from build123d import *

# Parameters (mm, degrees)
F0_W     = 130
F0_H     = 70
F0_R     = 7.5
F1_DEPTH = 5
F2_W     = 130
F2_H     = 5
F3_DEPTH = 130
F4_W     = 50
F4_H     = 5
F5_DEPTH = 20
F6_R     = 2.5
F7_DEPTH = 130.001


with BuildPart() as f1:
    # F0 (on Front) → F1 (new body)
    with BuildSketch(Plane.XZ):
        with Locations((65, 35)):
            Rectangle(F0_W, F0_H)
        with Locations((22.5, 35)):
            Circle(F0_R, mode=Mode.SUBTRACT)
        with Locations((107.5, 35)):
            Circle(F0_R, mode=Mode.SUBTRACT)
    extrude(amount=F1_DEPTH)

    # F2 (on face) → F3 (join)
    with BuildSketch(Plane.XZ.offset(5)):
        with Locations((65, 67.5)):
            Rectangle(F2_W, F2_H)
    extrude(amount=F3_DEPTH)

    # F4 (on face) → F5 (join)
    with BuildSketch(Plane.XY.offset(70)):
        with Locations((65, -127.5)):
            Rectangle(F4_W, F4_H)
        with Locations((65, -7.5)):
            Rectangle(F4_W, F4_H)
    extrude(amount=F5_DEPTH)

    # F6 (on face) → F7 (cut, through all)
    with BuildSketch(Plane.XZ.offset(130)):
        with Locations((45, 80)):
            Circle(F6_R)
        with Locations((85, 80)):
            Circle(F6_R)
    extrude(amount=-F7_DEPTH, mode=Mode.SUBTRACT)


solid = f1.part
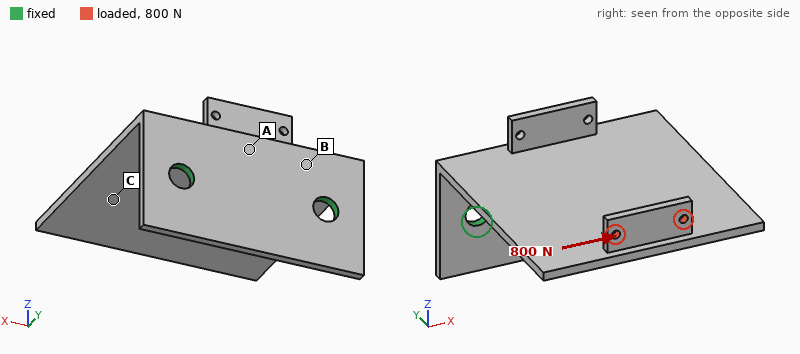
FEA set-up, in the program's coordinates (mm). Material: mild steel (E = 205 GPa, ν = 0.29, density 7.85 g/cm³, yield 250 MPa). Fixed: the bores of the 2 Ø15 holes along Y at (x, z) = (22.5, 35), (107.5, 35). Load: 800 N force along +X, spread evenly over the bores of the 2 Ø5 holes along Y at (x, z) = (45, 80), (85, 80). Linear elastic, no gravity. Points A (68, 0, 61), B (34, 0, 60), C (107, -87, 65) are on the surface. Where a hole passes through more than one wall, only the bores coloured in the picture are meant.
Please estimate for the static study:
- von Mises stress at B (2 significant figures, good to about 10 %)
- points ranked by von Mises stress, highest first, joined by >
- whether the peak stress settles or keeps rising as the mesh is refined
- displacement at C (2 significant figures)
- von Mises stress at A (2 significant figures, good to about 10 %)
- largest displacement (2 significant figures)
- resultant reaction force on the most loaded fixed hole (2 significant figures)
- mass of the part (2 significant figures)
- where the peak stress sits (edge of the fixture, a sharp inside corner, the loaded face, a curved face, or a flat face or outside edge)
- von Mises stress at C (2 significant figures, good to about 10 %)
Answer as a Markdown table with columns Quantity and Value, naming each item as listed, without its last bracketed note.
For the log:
| Quantity | Value |
|---|---|
| von Mises stress at B | 32 MPa |
| points ranked by von Mises stress, highest first, joined by > | B > A > C |
| whether the peak stress settles or keeps rising as the mesh is refined | keeps rising |
| displacement at C | 0.088 mm |
| von Mises stress at A | 19 MPa |
| largest displacement | 0.15 mm |
| resultant reaction force on the most loaded fixed hole | 1.2 kN |
| mass of the part | 1.1 kg |
| where the peak stress sits | edge of the fixture |
| von Mises stress at C | 9.3 MPa |
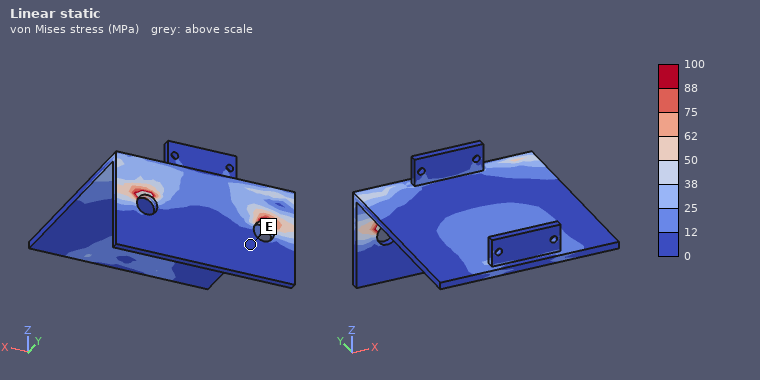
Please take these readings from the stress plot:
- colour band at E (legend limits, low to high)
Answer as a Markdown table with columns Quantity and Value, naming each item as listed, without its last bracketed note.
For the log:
| Quantity | Value |
|---|---|
| colour band at E | 0 to 12 MPa |
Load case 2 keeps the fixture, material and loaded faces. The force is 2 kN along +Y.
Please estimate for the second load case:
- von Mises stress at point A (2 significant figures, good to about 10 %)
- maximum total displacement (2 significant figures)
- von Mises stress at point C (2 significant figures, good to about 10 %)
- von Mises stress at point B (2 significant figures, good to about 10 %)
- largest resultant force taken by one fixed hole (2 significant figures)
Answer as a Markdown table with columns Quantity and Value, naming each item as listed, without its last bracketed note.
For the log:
| Quantity | Value |
|---|---|
| von Mises stress at point A | 70 MPa |
| maximum total displacement | 1.5 mm |
| von Mises stress at point C | 42 MPa |
| von Mises stress at point B | 70 MPa |
| largest resultant force taken by one fixed hole | 1.0 kN |
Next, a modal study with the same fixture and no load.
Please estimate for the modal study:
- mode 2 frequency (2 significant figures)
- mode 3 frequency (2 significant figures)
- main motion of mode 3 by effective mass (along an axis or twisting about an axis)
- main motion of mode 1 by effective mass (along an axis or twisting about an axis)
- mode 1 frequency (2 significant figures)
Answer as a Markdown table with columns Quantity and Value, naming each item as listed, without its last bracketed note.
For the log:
| Quantity | Value |
|---|---|
| mode 2 frequency | 510 Hz |
| mode 3 frequency | 730 Hz |
| main motion of mode 3 by effective mass | along X |
| main motion of mode 1 by effective mass | along Z |
| mode 1 frequency | 160 Hz |
